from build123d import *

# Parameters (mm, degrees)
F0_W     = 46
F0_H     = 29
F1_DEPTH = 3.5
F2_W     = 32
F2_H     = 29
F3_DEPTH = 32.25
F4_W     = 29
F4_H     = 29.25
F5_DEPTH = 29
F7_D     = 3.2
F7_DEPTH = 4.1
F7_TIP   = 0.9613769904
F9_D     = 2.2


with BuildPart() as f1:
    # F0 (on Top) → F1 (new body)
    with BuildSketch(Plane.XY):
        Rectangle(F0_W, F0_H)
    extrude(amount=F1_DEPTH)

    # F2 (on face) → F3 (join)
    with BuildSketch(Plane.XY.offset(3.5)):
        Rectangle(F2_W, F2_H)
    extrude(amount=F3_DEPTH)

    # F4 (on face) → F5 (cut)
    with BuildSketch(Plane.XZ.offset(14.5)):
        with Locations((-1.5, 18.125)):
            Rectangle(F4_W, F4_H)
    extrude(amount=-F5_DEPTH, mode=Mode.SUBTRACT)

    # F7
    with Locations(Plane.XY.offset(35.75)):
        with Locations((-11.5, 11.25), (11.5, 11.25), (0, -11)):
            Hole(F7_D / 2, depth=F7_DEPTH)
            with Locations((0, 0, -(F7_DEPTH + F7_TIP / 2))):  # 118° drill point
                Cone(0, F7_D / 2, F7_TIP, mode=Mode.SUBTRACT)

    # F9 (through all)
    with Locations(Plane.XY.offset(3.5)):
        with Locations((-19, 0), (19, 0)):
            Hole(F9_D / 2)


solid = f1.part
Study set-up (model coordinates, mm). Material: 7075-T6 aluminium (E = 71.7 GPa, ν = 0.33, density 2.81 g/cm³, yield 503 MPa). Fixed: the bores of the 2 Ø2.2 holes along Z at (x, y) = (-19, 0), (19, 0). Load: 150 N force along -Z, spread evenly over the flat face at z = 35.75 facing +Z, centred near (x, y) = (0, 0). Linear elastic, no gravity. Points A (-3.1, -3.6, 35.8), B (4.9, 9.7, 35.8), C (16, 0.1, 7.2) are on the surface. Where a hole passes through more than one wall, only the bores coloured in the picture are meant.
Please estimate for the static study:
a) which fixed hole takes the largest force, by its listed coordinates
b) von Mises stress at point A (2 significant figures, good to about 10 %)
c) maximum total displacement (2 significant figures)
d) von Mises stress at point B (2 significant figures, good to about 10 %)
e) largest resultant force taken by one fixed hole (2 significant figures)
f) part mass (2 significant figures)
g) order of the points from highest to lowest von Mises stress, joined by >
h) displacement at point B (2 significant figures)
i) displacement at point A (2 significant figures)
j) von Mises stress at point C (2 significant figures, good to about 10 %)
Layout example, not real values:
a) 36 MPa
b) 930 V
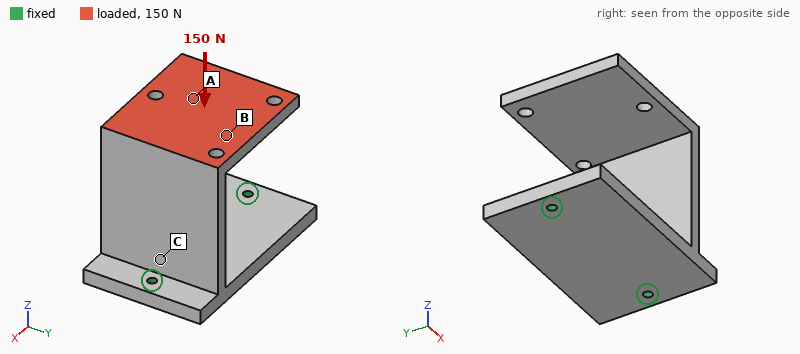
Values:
a) (19, 0)
b) 9.0 MPa
c) 0.63 mm
d) 21 MPa
e) 93 N
f) 28 g
g) C > B > A
h) 0.33 mm
i) 0.43 mm
j) 42 MPa
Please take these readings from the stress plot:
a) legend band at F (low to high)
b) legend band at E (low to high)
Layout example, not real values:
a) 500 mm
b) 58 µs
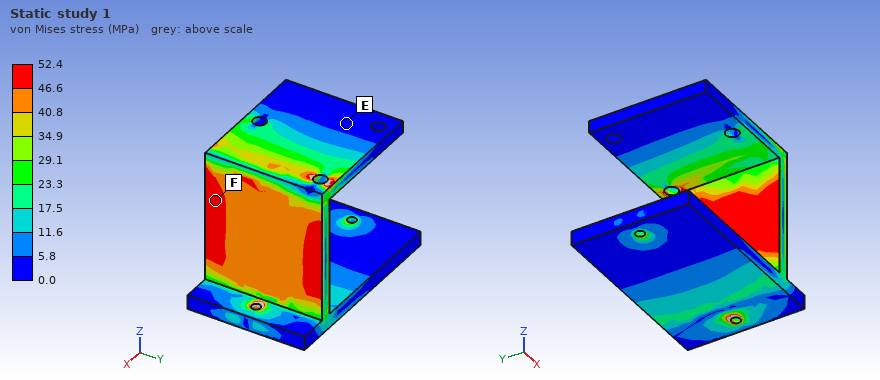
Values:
a) 46.6 to 52.4 MPa
b) 0.0 to 5.8 MPa
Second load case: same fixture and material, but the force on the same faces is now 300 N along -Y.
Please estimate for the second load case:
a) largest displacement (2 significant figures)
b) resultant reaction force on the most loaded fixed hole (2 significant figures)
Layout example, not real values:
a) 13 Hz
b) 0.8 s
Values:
a) 0.70 mm
b) 160 N
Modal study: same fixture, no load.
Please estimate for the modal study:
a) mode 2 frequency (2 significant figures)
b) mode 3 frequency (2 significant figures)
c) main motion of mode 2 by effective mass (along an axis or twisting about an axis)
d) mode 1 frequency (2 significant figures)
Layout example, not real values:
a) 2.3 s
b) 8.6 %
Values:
a) 1300 Hz
b) 2300 Hz
c) along Y
d) 810 Hz
